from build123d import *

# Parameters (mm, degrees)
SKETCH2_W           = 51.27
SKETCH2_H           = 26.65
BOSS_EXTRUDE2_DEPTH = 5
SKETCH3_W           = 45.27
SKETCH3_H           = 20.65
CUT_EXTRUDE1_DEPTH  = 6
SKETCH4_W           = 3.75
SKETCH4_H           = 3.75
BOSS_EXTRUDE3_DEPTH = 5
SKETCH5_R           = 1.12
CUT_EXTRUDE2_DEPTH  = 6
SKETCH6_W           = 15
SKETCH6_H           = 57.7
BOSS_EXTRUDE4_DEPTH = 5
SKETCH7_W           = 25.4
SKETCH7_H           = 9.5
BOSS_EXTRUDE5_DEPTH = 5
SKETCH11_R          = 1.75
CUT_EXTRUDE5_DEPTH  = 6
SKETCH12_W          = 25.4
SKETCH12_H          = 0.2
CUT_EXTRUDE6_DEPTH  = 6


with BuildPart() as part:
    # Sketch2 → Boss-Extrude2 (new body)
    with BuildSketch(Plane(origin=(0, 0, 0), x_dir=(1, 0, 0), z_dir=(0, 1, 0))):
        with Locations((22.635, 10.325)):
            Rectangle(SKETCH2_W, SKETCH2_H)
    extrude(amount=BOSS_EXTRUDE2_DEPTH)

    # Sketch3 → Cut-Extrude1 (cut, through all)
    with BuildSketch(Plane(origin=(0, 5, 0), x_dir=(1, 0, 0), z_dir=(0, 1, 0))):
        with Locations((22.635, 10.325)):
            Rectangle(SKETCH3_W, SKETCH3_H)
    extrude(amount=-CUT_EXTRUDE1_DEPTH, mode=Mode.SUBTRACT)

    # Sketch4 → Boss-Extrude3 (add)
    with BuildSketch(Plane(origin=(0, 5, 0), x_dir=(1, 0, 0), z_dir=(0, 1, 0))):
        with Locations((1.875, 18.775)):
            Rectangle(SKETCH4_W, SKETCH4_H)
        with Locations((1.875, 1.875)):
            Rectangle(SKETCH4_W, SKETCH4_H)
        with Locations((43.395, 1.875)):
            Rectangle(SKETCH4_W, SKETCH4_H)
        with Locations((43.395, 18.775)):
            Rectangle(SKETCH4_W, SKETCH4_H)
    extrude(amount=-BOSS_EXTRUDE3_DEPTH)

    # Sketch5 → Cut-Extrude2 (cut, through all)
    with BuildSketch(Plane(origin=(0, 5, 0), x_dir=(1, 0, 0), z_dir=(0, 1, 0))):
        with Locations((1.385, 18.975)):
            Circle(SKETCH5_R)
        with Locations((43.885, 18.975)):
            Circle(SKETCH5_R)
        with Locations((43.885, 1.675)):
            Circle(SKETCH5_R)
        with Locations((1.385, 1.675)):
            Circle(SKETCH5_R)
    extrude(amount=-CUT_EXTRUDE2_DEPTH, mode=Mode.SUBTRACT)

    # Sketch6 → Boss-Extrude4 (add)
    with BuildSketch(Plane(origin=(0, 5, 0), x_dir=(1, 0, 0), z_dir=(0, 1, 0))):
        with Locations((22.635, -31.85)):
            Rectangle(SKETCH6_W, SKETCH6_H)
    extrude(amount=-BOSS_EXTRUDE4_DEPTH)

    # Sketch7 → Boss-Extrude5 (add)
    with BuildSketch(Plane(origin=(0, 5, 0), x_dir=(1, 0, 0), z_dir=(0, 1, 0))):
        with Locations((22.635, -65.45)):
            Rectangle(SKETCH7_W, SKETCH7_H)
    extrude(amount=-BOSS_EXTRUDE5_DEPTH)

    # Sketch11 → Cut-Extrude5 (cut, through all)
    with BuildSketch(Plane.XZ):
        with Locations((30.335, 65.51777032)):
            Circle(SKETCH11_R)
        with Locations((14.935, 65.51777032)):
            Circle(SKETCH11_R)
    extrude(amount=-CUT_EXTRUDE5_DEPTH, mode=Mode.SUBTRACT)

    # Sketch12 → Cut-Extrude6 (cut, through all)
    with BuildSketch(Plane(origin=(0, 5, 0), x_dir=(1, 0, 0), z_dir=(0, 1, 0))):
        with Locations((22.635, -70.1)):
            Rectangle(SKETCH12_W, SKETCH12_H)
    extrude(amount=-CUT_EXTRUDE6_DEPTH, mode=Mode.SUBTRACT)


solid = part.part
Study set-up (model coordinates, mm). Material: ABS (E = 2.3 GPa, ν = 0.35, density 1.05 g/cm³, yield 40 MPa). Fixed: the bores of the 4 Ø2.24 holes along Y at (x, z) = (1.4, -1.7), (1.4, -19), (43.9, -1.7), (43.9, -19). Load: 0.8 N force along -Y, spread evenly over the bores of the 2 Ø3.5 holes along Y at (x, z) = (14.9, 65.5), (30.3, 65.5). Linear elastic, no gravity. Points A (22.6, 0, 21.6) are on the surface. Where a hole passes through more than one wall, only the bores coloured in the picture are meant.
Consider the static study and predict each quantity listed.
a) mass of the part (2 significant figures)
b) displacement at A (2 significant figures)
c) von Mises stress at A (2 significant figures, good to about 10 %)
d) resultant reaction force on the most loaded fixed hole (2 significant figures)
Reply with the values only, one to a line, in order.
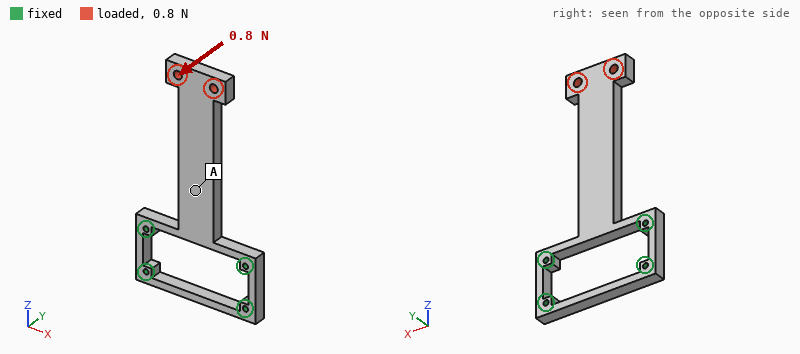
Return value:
8.2 g
0.30 mm
0.56 MPa
0.47 N
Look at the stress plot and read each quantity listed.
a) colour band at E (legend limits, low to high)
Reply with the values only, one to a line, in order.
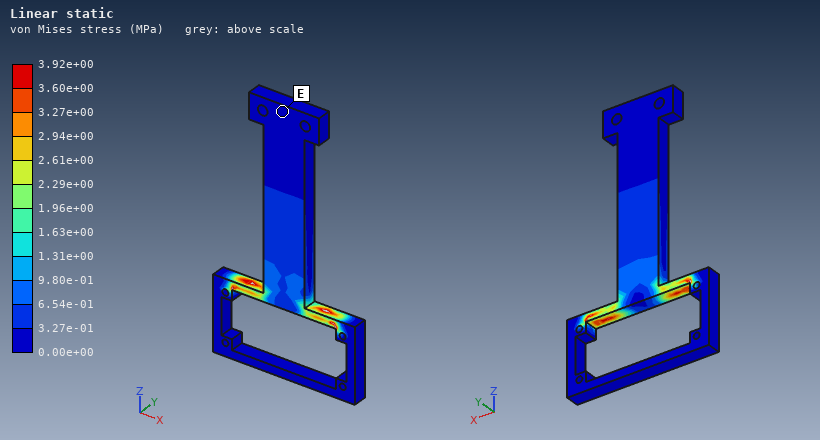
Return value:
0.00e+00 to 3.27e-01 MPa
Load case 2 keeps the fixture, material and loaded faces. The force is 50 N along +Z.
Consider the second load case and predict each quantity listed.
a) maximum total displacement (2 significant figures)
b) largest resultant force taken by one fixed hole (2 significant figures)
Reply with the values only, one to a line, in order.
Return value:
0.29 mm
42 N
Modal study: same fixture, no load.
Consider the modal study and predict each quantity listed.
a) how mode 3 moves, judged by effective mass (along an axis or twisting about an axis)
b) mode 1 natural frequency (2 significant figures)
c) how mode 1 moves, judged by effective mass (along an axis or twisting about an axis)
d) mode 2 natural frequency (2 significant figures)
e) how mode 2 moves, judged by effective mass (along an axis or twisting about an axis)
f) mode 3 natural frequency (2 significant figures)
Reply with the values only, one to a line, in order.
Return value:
along Z
90 Hz
along Y
280 Hz
along X
880 Hz
